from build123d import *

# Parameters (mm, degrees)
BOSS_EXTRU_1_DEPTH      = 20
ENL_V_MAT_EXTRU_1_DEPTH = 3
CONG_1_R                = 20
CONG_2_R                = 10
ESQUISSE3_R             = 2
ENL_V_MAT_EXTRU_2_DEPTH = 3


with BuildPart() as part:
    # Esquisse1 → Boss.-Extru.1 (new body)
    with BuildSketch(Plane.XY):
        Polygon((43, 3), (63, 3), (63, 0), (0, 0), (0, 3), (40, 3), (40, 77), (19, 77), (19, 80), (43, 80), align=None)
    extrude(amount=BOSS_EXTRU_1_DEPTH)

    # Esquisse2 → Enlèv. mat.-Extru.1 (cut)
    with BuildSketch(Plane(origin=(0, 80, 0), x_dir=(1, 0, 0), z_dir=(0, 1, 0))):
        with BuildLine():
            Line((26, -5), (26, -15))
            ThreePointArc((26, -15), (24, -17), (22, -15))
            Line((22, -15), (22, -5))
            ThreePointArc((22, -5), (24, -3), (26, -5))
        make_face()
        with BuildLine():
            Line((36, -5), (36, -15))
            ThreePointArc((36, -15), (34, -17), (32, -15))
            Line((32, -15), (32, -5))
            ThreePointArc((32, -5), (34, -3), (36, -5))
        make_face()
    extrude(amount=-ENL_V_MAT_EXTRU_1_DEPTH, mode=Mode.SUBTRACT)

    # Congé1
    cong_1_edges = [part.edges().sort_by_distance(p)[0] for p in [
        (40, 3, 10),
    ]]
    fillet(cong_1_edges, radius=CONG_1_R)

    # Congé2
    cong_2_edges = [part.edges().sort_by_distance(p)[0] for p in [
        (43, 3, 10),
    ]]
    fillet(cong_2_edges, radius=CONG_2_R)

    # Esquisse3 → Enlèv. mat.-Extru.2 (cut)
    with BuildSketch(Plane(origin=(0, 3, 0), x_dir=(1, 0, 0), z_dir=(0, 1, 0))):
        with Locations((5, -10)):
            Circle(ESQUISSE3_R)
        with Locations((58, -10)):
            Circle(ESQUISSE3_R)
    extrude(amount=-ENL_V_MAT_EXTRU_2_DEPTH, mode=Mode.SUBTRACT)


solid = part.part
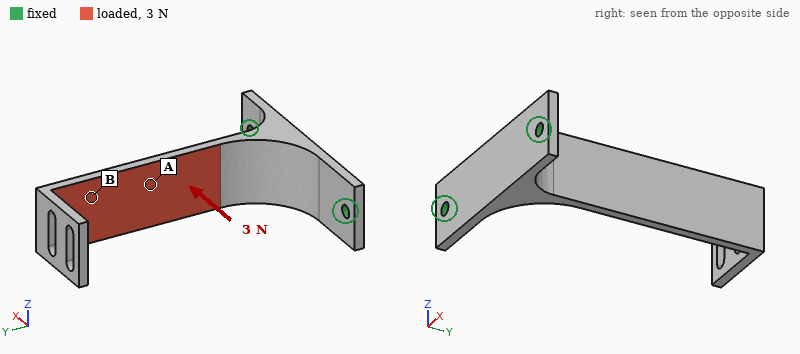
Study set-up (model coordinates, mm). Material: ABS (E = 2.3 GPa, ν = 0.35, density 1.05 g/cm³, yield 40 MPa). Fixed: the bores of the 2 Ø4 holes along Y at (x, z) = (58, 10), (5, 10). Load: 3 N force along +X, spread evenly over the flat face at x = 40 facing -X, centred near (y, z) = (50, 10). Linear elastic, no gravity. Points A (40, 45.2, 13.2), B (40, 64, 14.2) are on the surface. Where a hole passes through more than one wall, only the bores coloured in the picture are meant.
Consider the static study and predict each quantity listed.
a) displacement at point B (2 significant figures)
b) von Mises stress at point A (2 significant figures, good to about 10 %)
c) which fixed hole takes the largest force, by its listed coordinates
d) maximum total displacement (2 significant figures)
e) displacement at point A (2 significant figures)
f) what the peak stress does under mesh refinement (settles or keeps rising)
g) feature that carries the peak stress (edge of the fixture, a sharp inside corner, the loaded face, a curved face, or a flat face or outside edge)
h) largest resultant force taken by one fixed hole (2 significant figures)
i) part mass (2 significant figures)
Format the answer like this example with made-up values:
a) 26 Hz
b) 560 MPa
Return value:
a) 0.71 mm
b) 0.95 MPa
c) (5, 10)
d) 1.1 mm
e) 0.34 mm
f) keeps rising
g) edge of the fixture
h) 4.5 N
i) 12 g
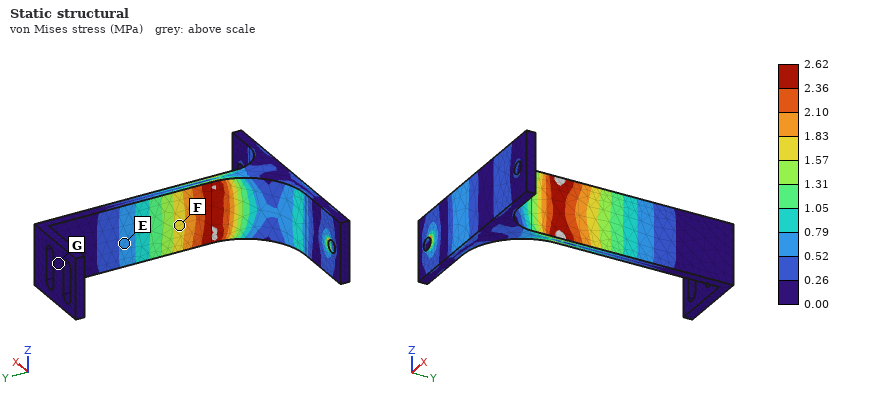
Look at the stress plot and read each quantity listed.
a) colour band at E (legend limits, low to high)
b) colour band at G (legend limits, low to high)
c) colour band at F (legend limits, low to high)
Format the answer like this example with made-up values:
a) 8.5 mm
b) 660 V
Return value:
a) 0.52 to 0.79 MPa
b) 0.00 to 0.26 MPa
c) 1.57 to 1.83 MPa
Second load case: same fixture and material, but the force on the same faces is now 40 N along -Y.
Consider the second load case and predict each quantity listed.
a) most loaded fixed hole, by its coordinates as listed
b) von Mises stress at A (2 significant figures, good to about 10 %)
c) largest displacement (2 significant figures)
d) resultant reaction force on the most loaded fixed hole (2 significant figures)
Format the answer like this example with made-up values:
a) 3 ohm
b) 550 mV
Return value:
a) (58, 10)
b) 1.6 MPa
c) 1.1 mm
d) 33 N
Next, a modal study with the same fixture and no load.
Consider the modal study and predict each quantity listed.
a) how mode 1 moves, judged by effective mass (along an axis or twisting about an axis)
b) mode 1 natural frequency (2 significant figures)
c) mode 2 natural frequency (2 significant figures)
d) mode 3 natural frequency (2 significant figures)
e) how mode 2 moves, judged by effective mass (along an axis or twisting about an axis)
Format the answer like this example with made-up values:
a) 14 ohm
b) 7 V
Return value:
a) along X
b) 120 Hz
c) 200 Hz
d) 540 Hz
e) along Z
